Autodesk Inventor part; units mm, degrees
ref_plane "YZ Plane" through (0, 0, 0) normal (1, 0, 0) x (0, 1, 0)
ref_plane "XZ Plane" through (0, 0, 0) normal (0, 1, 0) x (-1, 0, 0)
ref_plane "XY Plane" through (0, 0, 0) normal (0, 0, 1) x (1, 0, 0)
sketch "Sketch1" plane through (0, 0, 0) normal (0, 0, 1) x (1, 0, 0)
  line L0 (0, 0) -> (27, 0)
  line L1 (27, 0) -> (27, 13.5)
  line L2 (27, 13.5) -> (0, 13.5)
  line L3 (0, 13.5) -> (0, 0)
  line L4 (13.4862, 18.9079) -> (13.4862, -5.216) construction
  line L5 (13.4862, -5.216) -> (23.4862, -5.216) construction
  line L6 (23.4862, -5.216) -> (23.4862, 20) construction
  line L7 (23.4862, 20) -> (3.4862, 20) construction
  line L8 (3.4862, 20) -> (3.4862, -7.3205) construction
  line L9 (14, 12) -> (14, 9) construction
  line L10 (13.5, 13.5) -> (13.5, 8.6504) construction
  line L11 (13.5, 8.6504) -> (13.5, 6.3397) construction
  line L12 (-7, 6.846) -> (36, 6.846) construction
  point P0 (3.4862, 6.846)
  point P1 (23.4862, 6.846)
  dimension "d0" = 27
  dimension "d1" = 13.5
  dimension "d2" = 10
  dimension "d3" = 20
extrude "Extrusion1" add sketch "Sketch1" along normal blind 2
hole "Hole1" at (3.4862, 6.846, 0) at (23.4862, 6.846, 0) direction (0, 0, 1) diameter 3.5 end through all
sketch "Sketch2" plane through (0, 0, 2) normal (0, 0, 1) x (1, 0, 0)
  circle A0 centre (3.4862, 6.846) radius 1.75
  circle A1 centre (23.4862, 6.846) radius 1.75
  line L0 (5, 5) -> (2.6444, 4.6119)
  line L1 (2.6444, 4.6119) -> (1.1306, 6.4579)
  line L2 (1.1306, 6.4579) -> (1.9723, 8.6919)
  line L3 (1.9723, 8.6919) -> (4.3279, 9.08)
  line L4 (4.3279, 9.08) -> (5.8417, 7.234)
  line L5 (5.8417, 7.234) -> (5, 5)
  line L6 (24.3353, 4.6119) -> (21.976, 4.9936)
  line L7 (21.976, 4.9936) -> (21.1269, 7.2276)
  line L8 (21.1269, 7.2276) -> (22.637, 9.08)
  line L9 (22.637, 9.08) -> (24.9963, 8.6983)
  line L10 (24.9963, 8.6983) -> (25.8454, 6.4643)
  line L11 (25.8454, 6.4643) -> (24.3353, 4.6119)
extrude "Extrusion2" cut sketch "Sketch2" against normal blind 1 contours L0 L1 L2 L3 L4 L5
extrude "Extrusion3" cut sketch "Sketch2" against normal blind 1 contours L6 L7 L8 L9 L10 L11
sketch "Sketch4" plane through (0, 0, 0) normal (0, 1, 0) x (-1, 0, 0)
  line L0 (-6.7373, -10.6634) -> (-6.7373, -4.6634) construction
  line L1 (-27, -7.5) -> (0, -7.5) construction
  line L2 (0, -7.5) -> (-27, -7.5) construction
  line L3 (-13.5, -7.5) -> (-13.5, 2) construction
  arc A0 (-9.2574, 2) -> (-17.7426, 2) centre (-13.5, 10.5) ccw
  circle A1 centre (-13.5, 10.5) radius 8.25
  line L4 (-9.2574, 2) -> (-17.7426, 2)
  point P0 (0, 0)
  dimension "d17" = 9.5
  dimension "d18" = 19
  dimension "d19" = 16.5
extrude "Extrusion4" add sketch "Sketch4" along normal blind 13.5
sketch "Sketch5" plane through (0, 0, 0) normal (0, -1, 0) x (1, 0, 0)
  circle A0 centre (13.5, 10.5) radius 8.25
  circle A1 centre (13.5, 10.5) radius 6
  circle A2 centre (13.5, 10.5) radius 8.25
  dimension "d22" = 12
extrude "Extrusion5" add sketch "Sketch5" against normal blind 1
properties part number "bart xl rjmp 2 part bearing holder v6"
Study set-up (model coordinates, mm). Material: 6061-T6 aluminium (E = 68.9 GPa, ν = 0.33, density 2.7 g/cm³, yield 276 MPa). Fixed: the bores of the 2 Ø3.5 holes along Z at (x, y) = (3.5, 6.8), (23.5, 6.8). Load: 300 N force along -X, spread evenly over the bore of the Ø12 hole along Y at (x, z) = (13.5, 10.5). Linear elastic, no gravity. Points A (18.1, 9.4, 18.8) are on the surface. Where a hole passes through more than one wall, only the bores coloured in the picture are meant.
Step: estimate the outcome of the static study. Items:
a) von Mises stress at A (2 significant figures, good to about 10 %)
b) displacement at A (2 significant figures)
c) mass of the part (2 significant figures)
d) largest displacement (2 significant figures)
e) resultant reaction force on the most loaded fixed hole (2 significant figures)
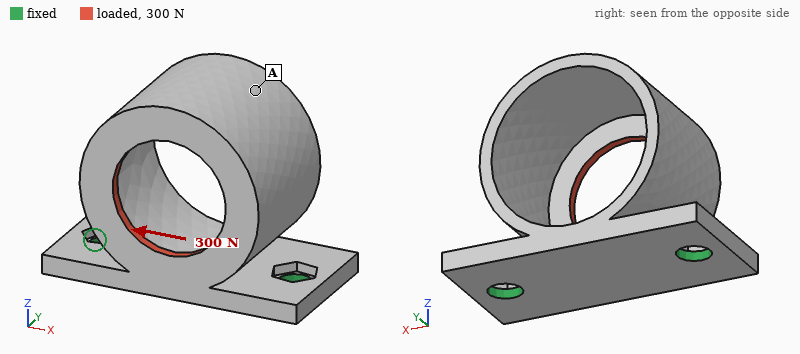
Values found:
23 MPa
0.16 mm
4.4 g
0.17 mm
260 N
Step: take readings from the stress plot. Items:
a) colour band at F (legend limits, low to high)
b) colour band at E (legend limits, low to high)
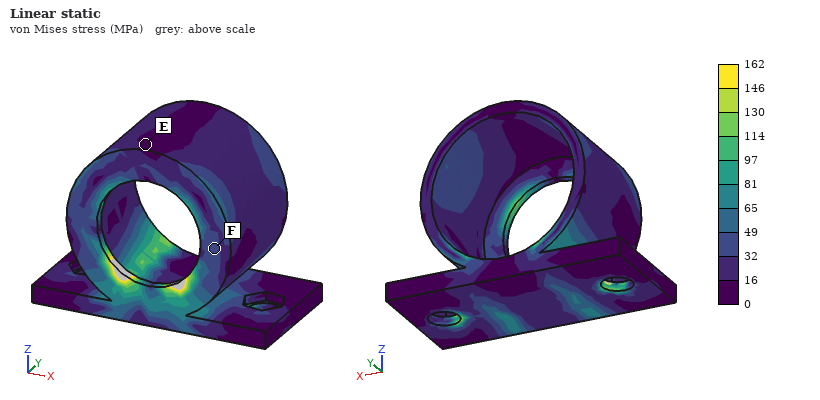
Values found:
32 to 49 MPa
0 to 16 MPa
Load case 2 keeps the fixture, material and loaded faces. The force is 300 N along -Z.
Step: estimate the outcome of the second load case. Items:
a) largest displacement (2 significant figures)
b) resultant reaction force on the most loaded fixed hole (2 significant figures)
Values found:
0.16 mm
210 N
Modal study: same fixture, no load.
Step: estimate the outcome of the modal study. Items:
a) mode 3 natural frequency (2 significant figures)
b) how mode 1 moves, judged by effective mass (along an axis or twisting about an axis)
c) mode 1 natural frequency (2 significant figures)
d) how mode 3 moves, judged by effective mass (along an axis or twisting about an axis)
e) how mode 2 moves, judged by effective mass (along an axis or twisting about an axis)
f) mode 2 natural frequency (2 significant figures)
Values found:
9600 Hz
along Y
3700 Hz
along Z
along X
4200 Hz
